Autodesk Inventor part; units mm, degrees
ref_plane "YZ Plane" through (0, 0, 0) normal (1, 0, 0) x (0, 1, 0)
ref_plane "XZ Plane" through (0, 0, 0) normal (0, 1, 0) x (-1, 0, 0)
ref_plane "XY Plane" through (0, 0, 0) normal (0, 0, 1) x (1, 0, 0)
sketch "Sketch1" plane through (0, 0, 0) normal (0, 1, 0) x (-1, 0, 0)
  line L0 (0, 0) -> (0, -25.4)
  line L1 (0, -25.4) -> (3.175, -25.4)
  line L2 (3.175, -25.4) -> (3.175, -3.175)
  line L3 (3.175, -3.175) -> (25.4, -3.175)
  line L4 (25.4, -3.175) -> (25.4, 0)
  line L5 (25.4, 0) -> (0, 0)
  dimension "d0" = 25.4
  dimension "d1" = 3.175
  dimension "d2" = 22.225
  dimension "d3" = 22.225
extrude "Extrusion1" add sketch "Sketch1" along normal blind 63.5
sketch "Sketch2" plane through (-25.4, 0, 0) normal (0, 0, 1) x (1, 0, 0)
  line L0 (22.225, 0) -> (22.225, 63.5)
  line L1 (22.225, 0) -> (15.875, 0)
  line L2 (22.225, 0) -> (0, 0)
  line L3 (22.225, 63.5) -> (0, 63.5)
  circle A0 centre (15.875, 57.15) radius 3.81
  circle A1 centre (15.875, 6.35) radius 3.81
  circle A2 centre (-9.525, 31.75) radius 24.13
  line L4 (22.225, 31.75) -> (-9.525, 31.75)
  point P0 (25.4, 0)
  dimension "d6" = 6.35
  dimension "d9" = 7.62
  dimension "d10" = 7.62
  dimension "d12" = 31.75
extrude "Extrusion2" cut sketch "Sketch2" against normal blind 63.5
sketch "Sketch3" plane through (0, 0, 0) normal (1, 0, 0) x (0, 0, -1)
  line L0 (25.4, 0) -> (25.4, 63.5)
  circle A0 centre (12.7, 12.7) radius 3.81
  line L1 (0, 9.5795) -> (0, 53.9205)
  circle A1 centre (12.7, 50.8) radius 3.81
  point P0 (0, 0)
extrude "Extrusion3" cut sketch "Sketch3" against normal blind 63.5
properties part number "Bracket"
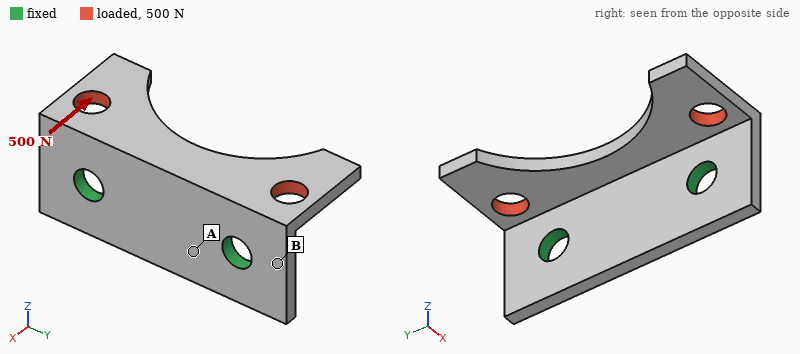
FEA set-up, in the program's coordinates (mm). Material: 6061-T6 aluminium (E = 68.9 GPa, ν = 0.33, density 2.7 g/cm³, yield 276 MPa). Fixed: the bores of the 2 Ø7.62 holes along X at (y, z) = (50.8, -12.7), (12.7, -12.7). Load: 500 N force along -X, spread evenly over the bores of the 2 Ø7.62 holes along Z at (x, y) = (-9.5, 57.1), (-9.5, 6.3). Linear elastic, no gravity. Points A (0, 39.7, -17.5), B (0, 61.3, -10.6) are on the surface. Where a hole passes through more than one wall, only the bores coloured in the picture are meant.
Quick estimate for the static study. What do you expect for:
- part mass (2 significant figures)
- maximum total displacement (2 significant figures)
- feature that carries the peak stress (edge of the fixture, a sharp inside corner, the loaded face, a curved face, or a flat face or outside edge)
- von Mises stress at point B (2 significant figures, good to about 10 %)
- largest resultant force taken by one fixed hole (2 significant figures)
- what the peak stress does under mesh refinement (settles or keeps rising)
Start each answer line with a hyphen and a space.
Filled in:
- 20 g
- 56 µm
- edge of the fixture
- 19 MPa
- 260 N
- keeps rising
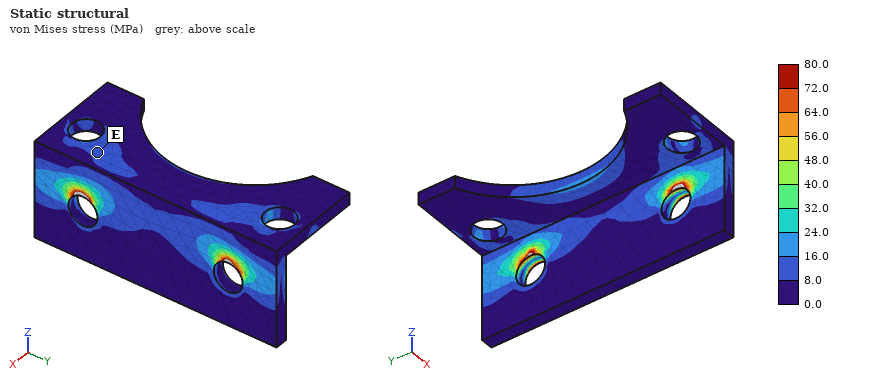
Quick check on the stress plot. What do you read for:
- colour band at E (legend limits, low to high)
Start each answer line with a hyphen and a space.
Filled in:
- 8.0 to 16.0 MPa
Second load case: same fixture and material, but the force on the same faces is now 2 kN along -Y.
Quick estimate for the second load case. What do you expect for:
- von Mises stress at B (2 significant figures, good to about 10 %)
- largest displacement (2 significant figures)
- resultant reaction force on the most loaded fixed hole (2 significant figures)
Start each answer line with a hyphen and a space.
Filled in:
- 39 MPa
- 76 µm
- 1.1 kN
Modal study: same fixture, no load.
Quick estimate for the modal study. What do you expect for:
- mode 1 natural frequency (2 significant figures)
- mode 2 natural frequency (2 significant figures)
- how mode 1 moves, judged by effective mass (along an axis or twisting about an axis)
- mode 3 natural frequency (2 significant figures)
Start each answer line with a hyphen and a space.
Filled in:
- 3800 Hz
- 4100 Hz
- along Z
- 9900 Hz
